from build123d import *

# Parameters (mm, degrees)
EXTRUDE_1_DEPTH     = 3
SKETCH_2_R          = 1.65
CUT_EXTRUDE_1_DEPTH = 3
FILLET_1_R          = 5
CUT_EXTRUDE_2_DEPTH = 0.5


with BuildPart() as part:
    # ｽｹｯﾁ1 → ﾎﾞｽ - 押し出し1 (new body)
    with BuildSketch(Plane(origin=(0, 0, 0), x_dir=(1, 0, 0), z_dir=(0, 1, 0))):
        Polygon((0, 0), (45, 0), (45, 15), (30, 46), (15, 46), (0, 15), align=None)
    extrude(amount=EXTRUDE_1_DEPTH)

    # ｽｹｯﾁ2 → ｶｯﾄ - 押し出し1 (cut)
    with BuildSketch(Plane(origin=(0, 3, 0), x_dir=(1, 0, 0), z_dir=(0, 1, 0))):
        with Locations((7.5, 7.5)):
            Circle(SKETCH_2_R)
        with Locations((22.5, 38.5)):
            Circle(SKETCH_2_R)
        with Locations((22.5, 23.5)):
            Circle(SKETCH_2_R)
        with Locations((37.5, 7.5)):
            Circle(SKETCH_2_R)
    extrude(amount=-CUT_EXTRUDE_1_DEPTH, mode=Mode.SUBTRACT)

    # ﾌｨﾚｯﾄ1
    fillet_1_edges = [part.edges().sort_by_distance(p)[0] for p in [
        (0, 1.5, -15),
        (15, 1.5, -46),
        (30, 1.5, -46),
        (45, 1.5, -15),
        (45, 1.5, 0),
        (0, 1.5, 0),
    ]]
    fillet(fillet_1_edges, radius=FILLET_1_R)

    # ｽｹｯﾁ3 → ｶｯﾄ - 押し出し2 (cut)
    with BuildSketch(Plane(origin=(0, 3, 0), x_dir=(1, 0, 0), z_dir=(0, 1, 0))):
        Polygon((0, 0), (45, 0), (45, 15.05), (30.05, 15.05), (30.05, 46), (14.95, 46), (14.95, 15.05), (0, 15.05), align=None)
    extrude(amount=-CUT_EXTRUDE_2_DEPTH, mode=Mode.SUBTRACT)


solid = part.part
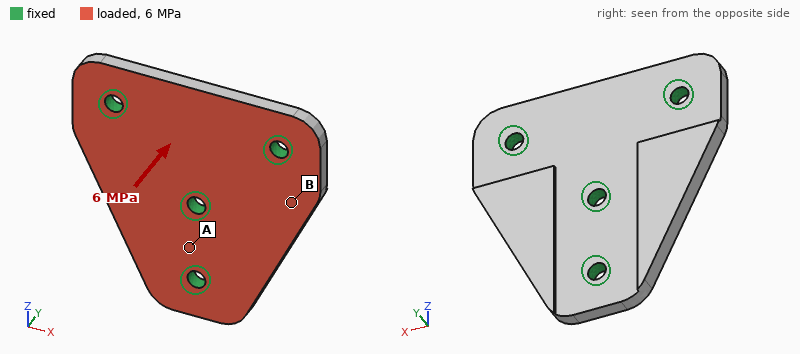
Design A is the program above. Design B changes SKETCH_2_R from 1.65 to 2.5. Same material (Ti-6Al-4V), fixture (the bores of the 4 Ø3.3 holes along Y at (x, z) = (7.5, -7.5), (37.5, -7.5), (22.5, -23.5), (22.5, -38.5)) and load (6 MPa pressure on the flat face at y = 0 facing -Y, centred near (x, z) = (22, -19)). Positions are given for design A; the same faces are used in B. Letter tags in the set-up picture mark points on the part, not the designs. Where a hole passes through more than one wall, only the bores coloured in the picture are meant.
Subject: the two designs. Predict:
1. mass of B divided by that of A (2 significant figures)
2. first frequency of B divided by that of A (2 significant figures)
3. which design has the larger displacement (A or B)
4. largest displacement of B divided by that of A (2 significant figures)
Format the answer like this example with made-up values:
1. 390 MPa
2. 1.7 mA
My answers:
1. 0.97
2. 1.2
3. A
4. 0.81
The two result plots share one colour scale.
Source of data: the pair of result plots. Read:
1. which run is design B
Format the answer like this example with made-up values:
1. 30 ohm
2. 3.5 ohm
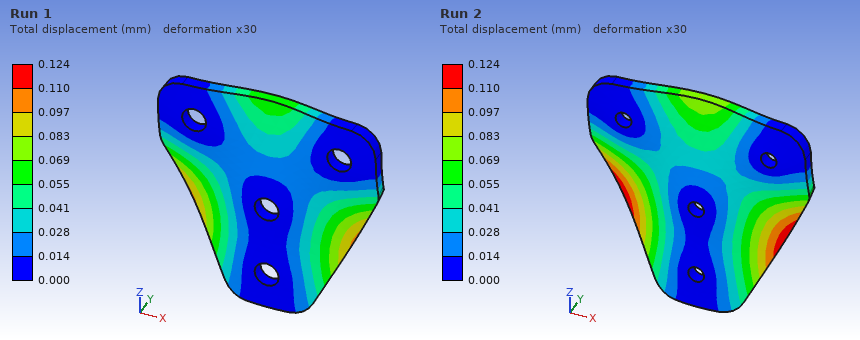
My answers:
1. Run 1
